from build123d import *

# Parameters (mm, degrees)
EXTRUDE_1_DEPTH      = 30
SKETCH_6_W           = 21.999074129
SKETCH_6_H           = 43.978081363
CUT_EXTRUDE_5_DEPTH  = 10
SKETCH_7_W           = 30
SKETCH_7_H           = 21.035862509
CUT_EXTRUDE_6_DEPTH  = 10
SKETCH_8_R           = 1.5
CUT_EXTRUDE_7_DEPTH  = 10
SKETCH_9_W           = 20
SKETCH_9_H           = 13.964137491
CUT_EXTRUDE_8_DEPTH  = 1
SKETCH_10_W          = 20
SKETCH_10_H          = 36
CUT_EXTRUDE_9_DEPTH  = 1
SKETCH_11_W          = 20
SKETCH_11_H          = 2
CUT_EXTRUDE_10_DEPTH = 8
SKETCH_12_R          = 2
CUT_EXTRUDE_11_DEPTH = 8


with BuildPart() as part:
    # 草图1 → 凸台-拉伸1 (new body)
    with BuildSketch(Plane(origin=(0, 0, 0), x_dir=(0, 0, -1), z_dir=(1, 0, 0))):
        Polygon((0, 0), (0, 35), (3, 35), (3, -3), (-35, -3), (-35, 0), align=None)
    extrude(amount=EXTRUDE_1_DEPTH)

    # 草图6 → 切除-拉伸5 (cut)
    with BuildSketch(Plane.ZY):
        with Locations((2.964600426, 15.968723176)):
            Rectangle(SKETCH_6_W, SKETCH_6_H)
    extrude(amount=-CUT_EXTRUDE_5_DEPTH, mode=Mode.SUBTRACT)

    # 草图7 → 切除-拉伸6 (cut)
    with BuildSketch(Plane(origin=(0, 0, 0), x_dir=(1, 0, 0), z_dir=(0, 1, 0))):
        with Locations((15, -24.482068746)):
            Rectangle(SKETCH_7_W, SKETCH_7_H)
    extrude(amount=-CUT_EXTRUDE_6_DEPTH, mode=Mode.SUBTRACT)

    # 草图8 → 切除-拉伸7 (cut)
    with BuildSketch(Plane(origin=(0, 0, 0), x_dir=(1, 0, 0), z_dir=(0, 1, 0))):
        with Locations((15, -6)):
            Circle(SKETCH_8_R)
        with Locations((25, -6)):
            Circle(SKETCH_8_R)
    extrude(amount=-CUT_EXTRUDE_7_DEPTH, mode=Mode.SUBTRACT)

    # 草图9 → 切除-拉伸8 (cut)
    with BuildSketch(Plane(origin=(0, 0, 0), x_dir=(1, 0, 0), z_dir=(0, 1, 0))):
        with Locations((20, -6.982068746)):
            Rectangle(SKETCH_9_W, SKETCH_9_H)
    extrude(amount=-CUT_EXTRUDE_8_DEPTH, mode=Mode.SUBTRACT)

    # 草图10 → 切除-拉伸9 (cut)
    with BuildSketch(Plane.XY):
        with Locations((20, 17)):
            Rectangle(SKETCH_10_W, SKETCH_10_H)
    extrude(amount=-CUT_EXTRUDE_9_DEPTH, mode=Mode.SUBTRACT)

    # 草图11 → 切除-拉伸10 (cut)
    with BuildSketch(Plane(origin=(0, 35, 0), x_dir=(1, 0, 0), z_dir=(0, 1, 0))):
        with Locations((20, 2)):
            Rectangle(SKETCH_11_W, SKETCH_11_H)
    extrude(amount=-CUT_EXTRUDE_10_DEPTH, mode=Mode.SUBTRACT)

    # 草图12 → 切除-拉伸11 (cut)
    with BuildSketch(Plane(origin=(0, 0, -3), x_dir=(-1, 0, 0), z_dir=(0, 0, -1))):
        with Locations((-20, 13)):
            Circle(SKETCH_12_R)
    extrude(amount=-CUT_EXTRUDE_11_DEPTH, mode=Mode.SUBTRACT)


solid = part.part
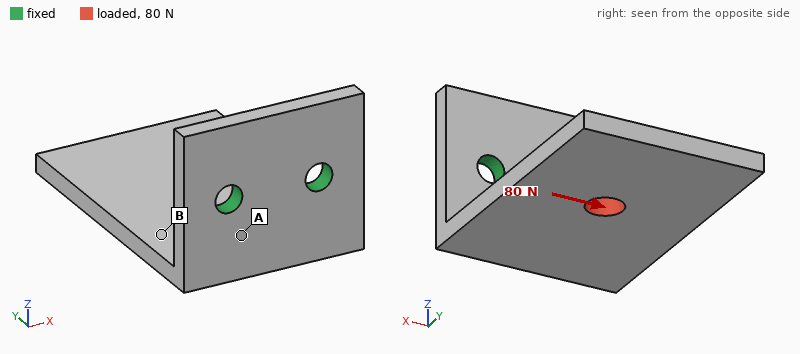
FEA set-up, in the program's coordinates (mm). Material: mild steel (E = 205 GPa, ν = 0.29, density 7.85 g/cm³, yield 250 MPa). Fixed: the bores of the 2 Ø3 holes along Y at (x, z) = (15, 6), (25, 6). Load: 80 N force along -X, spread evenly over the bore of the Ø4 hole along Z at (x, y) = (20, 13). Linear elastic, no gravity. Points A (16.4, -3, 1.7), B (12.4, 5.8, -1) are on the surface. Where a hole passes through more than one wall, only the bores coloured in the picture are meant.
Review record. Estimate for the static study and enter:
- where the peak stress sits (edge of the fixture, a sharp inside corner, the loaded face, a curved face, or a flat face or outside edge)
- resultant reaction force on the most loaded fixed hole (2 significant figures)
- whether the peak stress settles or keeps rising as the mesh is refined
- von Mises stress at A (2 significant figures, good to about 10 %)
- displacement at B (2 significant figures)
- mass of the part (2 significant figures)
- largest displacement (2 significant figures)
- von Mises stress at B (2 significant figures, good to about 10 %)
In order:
edge of the fixture
110 N
keeps rising
29 MPa
8.9 µm
14 g
24 µm
12 MPa
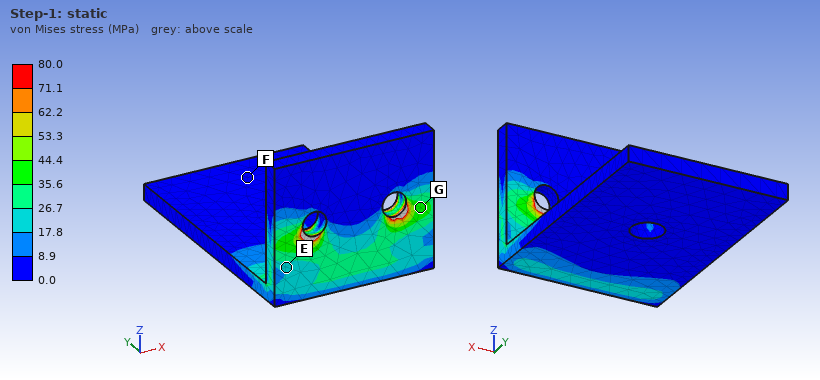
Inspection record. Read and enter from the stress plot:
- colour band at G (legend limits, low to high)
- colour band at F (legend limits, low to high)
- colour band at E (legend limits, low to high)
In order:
35.6 to 44.4 MPa
0.0 to 8.9 MPa
17.8 to 26.7 MPa
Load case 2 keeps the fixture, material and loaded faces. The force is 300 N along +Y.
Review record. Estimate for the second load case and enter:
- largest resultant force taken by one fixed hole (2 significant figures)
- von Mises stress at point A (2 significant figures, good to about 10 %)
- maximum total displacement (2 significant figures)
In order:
150 N
79 MPa
85 µm
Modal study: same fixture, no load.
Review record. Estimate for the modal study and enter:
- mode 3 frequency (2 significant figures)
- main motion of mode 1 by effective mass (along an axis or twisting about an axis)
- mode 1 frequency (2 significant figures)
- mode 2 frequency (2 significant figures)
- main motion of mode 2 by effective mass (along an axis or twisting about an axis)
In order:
6100 Hz
along Z
1400 Hz
3700 Hz
along X
